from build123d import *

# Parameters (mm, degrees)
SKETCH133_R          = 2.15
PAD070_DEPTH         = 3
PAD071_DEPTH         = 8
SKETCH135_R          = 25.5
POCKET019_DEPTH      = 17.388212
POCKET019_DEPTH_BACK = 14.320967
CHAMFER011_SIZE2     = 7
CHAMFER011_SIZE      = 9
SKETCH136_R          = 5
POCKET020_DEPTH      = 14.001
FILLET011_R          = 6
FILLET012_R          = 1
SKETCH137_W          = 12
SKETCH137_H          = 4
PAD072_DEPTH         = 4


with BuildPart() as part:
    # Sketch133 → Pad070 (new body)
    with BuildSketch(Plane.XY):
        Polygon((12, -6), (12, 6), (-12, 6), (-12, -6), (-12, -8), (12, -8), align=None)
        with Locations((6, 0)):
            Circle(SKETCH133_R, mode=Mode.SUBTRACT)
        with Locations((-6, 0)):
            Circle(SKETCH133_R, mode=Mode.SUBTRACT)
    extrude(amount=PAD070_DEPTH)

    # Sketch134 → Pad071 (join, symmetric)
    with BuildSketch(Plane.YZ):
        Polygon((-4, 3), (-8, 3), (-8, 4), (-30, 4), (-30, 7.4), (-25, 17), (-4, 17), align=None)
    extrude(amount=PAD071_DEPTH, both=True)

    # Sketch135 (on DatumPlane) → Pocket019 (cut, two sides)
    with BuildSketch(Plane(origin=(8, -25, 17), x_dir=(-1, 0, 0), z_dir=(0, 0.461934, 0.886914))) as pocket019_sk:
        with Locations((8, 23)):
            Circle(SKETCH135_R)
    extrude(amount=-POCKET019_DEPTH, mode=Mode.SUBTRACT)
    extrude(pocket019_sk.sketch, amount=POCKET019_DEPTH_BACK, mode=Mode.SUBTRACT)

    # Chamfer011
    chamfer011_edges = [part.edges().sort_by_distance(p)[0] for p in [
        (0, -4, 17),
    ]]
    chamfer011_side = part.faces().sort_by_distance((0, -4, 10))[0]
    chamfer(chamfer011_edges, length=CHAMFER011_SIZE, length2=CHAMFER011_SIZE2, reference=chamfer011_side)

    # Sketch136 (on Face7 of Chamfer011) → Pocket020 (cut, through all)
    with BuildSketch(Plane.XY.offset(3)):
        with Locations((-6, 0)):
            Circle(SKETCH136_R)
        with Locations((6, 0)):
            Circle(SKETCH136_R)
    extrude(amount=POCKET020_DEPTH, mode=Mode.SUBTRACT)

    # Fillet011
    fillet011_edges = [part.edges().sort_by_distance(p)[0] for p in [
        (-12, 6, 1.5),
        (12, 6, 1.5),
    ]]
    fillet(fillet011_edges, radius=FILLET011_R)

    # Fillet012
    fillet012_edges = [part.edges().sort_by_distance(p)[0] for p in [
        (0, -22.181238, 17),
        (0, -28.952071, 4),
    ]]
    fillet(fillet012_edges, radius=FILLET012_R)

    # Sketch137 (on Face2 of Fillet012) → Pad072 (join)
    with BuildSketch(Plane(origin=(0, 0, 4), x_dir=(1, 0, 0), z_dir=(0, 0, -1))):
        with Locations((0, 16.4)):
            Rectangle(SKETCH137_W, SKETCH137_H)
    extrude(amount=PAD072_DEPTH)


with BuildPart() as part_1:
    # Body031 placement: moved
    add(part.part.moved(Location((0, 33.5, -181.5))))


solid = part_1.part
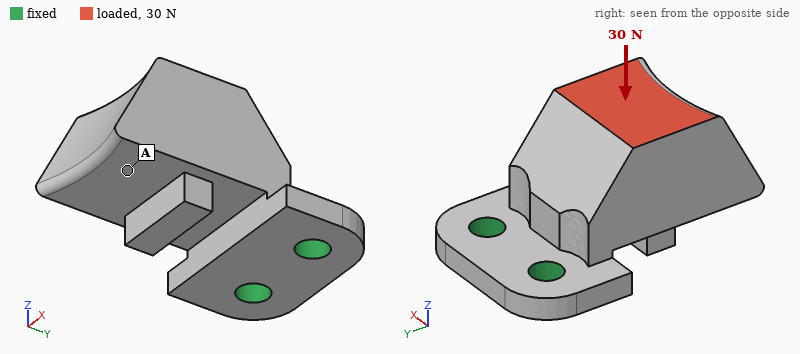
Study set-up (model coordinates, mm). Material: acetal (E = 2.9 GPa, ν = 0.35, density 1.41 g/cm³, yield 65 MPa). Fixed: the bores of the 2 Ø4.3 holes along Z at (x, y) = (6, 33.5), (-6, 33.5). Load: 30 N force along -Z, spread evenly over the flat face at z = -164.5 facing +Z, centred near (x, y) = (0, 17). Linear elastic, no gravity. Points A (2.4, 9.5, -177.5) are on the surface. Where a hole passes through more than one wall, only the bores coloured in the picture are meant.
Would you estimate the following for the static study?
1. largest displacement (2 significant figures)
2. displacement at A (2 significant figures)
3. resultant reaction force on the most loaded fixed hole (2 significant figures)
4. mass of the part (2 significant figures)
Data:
0.46 mm
0.36 mm
15 N
7.3 g
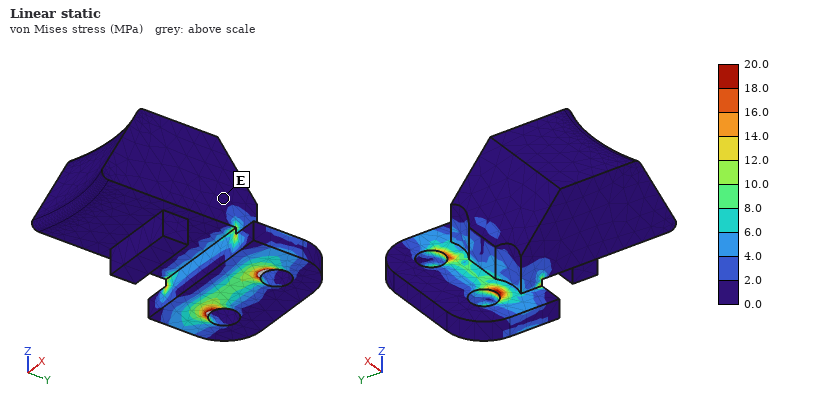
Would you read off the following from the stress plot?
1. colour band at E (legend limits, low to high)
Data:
0.0 to 2.0 MPa
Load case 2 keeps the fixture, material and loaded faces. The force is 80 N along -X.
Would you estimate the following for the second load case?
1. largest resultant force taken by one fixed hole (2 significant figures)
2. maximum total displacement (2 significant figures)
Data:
140 N
0.16 mm
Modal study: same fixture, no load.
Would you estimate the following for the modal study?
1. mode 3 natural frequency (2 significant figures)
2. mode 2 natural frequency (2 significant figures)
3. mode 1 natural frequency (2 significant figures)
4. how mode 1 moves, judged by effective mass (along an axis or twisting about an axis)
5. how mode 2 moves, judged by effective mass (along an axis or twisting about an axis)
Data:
3000 Hz
2000 Hz
600 Hz
along Z
along X
